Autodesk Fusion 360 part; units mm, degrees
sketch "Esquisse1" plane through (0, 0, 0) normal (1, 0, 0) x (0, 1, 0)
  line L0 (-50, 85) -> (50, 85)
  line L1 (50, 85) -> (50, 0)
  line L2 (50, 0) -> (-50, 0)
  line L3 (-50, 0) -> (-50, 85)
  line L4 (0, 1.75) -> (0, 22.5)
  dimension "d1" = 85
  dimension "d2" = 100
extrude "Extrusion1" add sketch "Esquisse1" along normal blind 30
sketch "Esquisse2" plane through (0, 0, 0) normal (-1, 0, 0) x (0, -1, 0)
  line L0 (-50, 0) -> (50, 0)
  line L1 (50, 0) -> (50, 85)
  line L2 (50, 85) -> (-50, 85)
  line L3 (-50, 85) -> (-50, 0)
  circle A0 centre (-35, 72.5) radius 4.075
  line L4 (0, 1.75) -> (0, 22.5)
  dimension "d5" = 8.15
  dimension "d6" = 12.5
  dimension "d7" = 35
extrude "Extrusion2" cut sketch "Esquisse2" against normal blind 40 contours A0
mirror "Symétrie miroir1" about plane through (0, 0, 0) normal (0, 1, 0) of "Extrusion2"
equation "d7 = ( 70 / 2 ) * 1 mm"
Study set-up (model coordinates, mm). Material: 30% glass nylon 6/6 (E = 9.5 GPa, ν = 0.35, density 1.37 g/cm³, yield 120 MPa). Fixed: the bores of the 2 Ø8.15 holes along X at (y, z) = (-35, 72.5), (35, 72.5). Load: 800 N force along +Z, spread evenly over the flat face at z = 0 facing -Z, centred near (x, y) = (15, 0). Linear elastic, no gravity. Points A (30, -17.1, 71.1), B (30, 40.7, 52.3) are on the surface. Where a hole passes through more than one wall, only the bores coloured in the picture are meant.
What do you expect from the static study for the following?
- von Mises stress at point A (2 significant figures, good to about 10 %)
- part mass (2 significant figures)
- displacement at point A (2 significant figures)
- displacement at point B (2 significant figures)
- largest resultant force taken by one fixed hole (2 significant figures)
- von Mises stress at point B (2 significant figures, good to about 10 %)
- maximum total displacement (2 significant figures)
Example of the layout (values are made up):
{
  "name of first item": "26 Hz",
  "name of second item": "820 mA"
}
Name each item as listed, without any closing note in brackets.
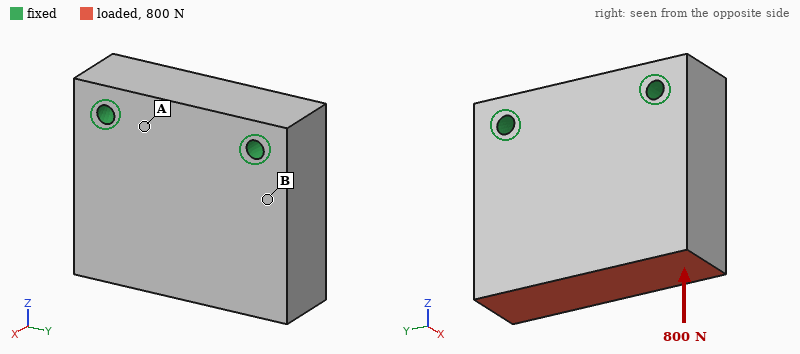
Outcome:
{
  "von Mises stress at point A": "0.16 MPa",
  "part mass": "350 g",
  "displacement at point A": "1.1 µm",
  "displacement at point B": "0.97 µm",
  "largest resultant force taken by one fixed hole": "410 N",
  "von Mises stress at point B": "0.36 MPa",
  "maximum total displacement": "2.6 µm"
}
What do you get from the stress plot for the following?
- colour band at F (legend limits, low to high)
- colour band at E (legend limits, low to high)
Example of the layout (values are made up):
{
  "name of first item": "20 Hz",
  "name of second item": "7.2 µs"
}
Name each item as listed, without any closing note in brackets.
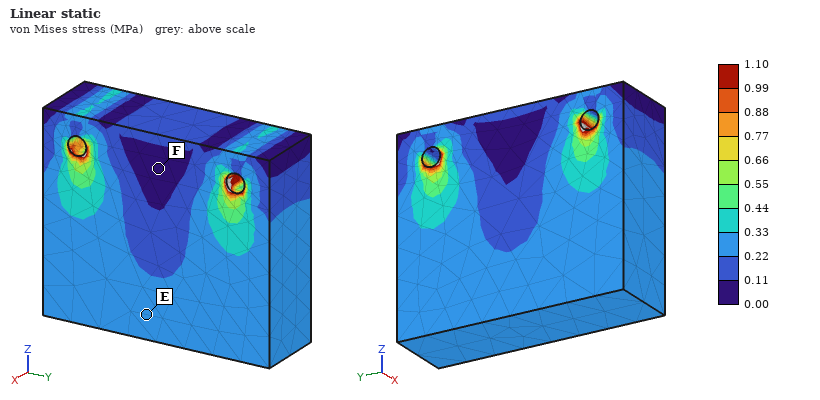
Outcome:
{
  "colour band at F": "0.00 to 0.11 MPa",
  "colour band at E": "0.22 to 0.33 MPa"
}
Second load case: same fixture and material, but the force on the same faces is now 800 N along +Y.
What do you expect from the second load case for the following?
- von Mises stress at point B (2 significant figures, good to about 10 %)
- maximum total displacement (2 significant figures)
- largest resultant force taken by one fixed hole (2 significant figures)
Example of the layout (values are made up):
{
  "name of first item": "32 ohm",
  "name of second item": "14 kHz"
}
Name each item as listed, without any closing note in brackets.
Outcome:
{
  "von Mises stress at point B": "0.69 MPa",
  "maximum total displacement": "15 µm",
  "largest resultant force taken by one fixed hole": "880 N"
}
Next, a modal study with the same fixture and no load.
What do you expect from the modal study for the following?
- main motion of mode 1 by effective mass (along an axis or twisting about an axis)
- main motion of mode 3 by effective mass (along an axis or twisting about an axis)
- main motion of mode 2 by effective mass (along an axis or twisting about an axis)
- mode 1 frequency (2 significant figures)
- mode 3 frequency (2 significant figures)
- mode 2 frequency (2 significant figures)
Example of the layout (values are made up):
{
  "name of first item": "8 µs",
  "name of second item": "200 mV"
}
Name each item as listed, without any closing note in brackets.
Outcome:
{
  "main motion of mode 1 by effective mass": "along X",
  "main motion of mode 3 by effective mass": "along Y",
  "main motion of mode 2 by effective mass": "twisting about Z",
  "mode 1 frequency": "1800 Hz",
  "mode 3 frequency": "3900 Hz",
  "mode 2 frequency": "3500 Hz"
}
